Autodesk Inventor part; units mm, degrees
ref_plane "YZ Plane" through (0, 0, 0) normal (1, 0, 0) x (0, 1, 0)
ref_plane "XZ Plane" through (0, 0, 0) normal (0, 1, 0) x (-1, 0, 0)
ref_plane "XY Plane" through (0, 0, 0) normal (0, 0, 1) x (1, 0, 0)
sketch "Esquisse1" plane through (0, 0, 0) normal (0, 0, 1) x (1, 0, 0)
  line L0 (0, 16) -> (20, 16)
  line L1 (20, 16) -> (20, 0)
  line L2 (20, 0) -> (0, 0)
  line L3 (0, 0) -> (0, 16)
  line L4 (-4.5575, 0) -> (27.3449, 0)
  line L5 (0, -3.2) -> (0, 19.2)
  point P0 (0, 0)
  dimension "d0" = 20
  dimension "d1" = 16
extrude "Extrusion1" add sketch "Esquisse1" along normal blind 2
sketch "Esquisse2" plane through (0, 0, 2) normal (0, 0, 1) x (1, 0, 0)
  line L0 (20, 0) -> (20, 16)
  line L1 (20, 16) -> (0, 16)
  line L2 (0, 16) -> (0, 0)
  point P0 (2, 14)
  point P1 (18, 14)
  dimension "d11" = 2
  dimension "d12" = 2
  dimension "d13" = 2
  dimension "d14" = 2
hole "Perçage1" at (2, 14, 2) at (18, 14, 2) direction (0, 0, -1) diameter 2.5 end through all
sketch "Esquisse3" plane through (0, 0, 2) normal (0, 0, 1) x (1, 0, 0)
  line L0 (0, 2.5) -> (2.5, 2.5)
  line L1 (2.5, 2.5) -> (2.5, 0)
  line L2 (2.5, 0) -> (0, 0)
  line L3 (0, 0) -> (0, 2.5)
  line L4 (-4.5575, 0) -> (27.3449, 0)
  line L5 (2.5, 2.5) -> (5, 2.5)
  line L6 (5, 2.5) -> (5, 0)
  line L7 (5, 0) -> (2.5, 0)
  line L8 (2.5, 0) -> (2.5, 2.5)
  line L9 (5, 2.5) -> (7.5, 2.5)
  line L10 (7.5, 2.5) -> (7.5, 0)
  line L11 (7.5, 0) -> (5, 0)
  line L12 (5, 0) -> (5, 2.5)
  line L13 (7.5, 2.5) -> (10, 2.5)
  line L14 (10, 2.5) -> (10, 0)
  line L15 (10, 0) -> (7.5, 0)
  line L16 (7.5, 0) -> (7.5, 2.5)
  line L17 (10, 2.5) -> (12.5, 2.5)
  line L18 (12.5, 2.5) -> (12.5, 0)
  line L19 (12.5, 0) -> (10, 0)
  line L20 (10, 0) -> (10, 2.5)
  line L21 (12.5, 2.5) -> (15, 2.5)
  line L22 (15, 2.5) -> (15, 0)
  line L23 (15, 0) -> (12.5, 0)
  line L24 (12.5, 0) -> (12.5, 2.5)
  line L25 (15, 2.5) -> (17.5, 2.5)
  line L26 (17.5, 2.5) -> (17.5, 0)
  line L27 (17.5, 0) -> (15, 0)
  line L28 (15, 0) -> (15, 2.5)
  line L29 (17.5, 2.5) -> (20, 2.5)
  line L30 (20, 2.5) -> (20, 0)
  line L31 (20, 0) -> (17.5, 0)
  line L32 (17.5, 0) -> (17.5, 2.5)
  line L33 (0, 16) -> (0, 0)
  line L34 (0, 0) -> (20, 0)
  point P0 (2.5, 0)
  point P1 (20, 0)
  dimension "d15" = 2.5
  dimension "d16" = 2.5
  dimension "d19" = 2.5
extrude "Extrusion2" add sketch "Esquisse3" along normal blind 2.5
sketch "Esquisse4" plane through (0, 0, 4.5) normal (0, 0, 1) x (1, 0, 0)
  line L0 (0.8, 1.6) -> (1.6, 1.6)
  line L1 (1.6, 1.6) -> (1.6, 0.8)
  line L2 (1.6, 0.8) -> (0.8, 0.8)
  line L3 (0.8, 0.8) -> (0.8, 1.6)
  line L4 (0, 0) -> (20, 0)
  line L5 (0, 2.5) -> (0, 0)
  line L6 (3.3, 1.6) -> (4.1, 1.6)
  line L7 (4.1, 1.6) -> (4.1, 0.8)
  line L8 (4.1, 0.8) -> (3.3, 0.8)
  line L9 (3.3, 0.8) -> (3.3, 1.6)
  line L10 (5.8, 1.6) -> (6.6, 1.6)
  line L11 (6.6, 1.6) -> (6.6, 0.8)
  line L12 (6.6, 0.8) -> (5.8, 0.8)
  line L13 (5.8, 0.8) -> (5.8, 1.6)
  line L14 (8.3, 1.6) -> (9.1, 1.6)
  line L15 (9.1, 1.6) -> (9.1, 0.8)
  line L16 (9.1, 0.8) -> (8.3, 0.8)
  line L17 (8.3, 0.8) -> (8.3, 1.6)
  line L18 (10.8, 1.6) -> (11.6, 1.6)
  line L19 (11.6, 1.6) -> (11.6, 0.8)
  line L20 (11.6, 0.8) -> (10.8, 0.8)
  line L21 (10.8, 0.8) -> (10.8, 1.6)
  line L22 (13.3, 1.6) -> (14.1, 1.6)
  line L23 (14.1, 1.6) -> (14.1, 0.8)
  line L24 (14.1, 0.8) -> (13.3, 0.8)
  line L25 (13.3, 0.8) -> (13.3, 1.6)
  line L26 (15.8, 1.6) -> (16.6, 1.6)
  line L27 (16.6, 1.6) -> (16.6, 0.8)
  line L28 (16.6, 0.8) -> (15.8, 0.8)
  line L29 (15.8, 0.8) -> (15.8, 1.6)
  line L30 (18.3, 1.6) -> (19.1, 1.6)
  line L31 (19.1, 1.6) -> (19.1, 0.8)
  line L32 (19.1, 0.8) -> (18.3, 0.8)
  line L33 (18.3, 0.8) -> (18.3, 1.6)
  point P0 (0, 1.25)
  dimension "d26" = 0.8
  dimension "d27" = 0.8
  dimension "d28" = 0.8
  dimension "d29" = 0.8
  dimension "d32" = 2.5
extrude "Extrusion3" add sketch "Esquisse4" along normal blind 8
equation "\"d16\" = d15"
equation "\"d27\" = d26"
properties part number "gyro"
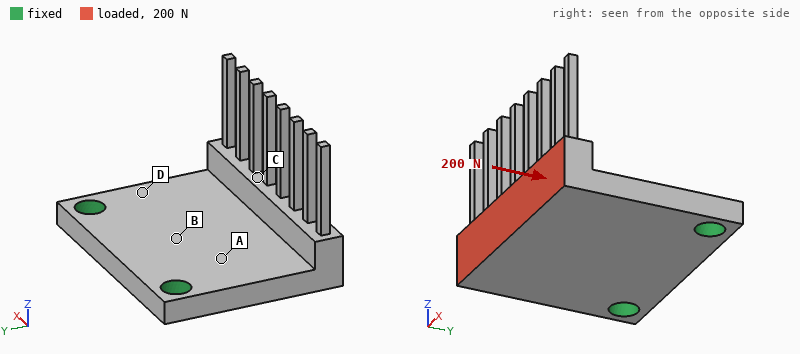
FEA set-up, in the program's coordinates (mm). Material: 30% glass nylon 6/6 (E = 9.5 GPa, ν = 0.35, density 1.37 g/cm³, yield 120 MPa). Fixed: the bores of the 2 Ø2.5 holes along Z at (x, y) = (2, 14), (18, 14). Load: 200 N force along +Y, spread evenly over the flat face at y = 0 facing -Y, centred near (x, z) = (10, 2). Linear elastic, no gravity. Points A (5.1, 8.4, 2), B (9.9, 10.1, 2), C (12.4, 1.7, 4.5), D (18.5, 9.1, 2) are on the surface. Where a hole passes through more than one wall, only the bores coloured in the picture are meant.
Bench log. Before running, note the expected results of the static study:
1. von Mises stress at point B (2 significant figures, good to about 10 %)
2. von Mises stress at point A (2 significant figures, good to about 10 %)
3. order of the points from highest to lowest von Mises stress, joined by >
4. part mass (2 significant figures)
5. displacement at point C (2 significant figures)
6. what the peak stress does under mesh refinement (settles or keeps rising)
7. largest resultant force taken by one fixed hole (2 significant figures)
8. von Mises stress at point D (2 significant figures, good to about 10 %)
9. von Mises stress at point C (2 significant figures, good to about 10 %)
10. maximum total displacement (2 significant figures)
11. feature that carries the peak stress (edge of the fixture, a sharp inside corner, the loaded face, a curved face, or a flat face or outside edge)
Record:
15 MPa
22 MPa
D > A > B > C
1.1 g
0.18 mm
keeps rising
100 N
28 MPa
4.0 MPa
0.34 mm
edge of the fixture
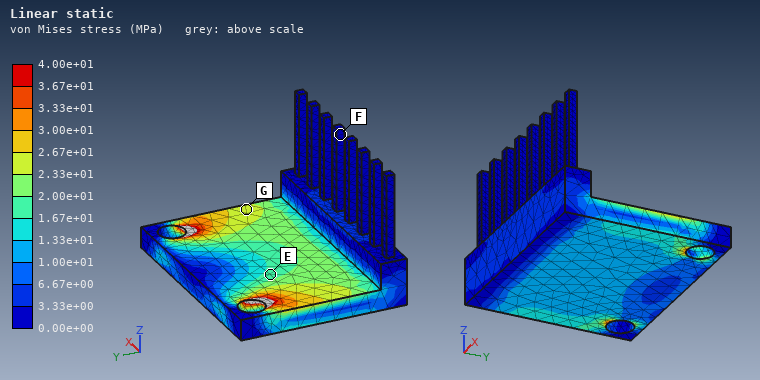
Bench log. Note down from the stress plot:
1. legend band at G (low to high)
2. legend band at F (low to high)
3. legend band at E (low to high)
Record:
2.33e+01 to 2.67e+01 MPa
0.00e+00 to 3.33e+00 MPa
1.67e+01 to 2.00e+01 MPa
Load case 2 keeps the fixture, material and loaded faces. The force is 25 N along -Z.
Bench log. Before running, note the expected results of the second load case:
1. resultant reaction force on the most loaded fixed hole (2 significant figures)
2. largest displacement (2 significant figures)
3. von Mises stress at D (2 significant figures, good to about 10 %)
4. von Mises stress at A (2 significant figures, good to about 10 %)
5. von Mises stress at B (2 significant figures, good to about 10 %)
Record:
13 N
0.29 mm
20 MPa
15 MPa
12 MPa
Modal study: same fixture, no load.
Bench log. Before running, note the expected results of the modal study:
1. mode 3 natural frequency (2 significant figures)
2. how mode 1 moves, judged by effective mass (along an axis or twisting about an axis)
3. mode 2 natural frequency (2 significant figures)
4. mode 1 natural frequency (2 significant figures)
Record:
5000 Hz
along Z
4600 Hz
2800 Hz
